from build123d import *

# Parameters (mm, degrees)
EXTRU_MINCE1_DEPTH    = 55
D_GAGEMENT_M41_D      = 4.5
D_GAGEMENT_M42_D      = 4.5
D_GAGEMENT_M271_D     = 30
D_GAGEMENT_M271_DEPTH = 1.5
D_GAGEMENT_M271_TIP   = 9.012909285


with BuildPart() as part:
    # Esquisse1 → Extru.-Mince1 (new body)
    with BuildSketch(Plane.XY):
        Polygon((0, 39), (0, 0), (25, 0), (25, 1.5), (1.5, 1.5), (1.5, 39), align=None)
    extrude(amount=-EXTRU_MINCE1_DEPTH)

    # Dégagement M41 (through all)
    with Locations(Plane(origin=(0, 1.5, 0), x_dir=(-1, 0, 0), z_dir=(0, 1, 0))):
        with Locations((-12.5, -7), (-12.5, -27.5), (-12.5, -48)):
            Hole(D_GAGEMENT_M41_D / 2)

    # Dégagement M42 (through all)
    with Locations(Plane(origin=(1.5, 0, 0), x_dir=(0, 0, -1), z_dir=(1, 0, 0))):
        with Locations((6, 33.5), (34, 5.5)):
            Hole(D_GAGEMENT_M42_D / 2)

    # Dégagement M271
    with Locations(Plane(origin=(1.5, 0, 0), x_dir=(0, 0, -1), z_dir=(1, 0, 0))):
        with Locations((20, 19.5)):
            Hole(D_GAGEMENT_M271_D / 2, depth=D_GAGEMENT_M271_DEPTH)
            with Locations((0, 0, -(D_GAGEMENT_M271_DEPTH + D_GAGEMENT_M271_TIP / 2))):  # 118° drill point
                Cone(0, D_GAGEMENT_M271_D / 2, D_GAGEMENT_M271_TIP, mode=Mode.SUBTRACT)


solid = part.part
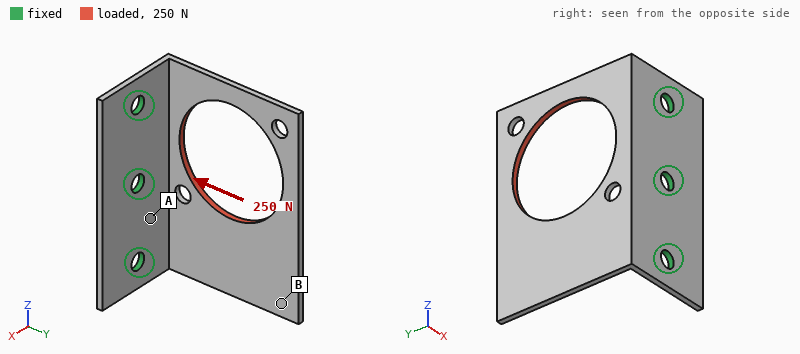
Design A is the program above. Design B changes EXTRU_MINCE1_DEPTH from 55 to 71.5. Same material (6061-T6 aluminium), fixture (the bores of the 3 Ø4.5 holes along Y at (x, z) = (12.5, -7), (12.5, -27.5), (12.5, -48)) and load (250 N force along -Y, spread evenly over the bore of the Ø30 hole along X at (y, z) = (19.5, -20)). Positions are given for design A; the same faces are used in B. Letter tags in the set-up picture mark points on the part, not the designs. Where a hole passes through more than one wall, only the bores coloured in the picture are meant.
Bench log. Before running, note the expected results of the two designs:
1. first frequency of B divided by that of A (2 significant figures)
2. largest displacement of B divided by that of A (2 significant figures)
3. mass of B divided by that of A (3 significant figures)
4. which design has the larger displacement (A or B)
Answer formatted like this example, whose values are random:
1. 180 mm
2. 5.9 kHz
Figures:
1. 0.97
2. 0.92
3. 1.39
4. A
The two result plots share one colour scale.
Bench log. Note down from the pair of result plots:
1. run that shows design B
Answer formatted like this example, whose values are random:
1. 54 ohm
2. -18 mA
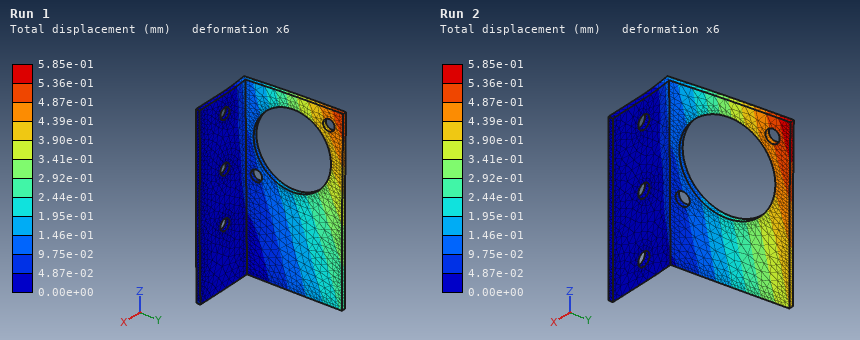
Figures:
1. Run 1
